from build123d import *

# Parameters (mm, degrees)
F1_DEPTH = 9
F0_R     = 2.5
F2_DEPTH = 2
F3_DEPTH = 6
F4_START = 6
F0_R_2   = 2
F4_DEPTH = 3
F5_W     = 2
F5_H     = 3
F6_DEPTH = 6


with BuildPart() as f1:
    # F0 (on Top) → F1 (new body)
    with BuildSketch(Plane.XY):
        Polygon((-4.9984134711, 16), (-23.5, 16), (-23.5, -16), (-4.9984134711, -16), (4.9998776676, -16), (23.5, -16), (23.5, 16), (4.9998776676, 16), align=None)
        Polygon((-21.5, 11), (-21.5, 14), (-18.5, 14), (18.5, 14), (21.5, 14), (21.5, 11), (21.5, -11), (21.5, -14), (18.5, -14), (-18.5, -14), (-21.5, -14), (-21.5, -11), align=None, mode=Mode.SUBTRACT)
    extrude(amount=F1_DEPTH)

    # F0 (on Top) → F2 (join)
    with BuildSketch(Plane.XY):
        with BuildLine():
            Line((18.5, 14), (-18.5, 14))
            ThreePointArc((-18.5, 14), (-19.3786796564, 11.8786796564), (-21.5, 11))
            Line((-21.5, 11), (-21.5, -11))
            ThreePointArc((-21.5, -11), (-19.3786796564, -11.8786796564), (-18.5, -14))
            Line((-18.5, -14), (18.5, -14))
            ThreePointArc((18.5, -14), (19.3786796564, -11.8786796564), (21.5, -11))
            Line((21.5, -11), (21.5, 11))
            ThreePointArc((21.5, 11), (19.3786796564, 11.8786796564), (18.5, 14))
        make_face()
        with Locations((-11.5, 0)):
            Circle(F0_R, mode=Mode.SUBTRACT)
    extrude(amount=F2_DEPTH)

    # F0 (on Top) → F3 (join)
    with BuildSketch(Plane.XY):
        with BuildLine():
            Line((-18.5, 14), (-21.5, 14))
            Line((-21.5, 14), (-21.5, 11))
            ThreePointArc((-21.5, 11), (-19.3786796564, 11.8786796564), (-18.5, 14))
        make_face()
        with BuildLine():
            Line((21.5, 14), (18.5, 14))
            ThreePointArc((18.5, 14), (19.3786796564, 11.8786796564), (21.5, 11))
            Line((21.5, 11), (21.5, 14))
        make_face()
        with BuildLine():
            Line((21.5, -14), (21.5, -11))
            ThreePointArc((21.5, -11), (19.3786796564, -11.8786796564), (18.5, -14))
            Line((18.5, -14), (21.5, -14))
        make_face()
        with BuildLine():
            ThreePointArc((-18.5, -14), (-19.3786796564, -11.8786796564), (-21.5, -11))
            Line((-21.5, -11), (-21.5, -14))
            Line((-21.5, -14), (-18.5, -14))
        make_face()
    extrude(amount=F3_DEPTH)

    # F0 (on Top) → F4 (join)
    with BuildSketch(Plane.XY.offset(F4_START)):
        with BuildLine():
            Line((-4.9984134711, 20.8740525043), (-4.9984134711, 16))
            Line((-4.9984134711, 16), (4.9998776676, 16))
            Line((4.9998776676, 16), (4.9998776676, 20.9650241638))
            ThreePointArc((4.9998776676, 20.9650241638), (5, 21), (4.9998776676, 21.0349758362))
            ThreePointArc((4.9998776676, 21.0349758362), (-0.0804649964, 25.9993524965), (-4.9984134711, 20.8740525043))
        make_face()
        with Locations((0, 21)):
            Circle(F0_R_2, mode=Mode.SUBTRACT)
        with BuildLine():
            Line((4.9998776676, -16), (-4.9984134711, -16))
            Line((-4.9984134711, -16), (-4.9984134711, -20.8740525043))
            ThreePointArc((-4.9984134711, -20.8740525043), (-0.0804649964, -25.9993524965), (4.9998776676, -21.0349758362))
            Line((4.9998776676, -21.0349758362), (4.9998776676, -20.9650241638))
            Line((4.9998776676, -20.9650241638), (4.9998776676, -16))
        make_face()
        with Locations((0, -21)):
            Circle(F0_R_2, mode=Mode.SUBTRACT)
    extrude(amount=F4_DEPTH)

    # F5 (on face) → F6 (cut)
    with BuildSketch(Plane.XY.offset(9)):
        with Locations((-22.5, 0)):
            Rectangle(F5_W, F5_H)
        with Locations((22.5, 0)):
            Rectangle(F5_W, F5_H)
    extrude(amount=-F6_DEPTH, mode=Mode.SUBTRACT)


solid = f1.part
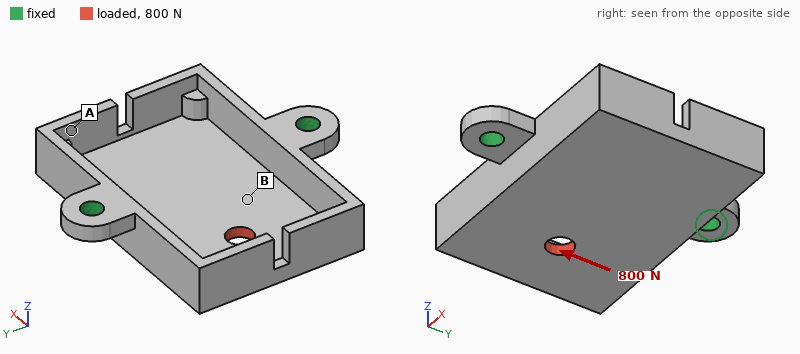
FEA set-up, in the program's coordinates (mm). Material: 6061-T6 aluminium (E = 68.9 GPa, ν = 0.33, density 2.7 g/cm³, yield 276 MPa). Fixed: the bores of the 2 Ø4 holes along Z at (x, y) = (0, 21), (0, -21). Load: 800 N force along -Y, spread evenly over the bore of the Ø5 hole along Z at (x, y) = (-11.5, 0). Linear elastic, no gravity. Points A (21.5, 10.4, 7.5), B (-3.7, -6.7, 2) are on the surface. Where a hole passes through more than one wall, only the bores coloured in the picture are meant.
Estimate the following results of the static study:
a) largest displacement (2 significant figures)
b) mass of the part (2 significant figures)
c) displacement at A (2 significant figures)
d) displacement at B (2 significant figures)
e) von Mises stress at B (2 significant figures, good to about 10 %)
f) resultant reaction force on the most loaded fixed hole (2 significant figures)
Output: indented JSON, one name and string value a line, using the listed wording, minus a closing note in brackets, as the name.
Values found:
{
  "largest displacement": "79 µm",
  "mass of the part": "15 g",
  "displacement at A": "15 µm",
  "displacement at B": "35 µm",
  "von Mises stress at B": "35 MPa",
  "resultant reaction force on the most loaded fixed hole": "480 N"
}
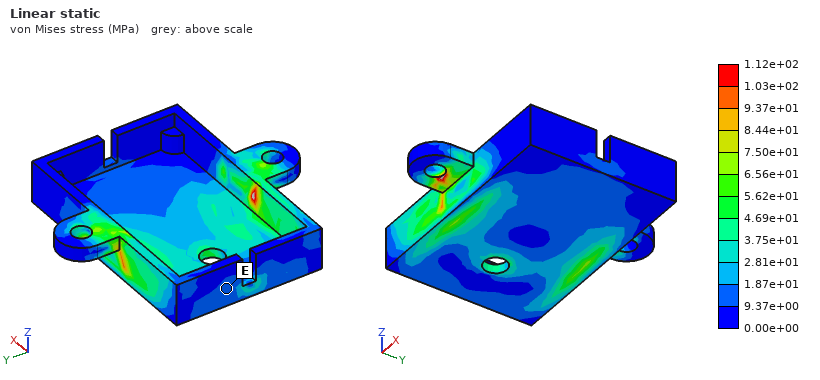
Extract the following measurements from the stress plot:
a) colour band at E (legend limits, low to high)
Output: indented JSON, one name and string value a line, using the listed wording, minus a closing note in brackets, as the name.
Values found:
{
  "colour band at E": "9.37e+00 to 1.87e+01 MPa"
}
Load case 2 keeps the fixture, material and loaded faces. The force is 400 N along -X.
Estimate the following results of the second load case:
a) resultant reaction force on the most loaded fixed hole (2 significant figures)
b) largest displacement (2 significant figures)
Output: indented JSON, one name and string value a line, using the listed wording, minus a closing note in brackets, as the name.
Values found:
{
  "resultant reaction force on the most loaded fixed hole": "200 N",
  "largest displacement": "66 µm"
}
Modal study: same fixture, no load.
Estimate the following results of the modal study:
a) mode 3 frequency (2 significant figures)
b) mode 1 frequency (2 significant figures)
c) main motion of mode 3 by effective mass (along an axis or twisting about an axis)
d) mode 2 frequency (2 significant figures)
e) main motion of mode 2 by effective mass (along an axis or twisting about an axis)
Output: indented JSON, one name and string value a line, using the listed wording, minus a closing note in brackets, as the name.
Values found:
{
  "mode 3 frequency": "6200 Hz",
  "mode 1 frequency": "2600 Hz",
  "main motion of mode 3 by effective mass": "along Z",
  "mode 2 frequency": "4600 Hz",
  "main motion of mode 2 by effective mass": "twisting about Z"
}
